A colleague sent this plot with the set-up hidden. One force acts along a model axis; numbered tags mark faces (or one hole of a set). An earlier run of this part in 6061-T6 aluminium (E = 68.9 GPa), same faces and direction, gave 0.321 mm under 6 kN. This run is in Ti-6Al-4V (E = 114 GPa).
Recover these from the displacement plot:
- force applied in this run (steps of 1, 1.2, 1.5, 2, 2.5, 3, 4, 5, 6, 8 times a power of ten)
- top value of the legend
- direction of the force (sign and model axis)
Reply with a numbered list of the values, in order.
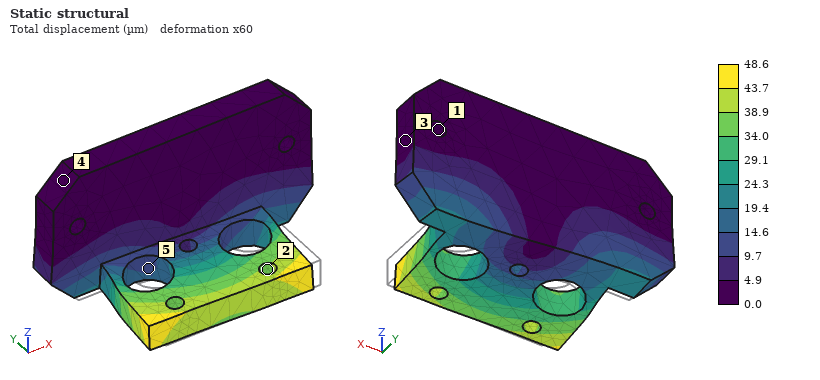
1. 1.5 kN
2. 48.6 µm
3. -X
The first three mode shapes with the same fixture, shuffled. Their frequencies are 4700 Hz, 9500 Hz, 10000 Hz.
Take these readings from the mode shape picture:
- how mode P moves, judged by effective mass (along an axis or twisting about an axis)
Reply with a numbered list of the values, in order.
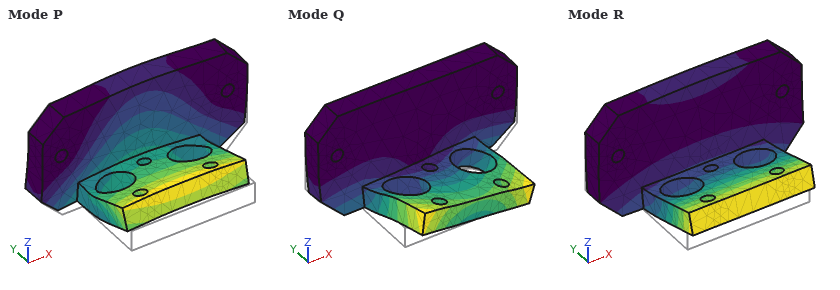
1. along Y
